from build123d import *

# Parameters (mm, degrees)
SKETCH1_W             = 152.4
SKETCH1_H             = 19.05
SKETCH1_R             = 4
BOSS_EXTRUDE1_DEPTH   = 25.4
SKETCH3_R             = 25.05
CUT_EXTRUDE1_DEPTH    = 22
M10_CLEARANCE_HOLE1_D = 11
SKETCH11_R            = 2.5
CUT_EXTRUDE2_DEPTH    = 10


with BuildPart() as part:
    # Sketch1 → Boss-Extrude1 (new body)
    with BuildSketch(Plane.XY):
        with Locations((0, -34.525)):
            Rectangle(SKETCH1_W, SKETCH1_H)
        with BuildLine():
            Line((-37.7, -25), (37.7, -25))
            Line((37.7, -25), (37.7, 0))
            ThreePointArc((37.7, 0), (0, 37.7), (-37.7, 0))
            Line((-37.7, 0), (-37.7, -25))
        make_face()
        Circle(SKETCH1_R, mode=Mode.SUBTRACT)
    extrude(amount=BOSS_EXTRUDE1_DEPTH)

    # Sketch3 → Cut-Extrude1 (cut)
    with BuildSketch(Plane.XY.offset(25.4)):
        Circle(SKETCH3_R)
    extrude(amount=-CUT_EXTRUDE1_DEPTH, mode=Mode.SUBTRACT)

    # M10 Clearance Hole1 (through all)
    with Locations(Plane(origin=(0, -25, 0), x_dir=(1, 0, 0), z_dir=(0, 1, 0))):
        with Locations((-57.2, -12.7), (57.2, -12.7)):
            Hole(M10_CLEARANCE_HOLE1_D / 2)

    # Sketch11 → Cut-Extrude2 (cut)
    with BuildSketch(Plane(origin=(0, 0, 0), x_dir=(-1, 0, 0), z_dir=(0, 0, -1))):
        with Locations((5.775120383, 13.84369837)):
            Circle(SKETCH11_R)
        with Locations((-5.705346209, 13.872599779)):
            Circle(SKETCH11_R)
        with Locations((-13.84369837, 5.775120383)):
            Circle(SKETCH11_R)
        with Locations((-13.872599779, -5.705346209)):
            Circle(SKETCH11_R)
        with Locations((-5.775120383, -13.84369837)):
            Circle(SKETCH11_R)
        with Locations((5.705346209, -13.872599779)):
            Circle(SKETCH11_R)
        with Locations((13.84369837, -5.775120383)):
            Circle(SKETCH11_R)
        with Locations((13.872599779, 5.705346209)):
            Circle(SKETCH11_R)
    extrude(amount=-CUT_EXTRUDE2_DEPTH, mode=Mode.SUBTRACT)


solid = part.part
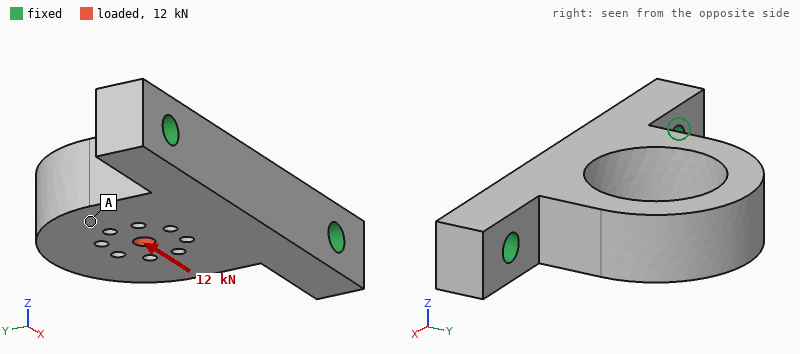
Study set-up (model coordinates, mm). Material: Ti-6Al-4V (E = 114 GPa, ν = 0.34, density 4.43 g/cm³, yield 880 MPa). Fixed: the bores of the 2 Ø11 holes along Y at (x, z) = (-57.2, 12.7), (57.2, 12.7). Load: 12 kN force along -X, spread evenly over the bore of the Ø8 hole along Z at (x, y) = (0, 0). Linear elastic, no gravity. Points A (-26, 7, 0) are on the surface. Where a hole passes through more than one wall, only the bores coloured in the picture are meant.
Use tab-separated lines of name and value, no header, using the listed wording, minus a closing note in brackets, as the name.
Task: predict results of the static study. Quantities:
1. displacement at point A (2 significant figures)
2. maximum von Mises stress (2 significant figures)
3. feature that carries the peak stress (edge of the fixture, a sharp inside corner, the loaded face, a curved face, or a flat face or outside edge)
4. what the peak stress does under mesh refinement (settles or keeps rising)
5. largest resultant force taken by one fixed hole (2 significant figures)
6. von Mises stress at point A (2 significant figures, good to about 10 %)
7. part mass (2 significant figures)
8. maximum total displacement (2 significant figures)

displacement at point A	32 µm
maximum von Mises stress	260 MPa
feature that carries the peak stress	a curved face
what the peak stress does under mesh refinement	settles
largest resultant force taken by one fixed hole	7.6 kN
von Mises stress at point A	20 MPa
part mass	580 g
maximum total displacement	48 µm
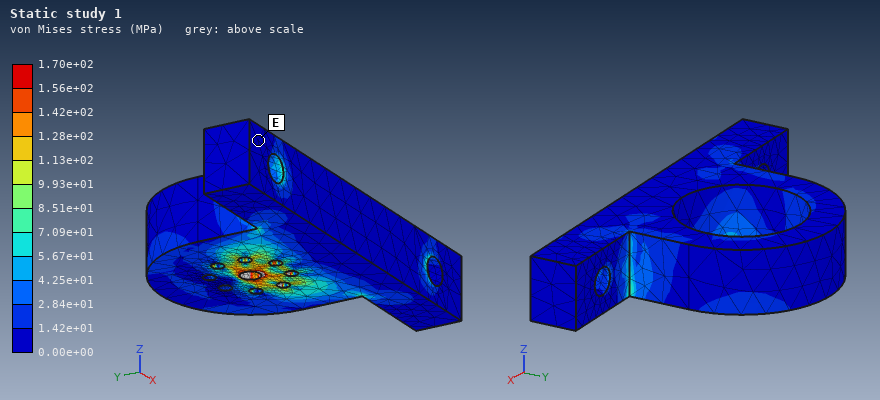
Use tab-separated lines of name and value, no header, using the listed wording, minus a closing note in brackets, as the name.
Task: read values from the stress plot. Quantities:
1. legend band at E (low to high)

legend band at E	0.00e+00 to 1.42e+01 MPa
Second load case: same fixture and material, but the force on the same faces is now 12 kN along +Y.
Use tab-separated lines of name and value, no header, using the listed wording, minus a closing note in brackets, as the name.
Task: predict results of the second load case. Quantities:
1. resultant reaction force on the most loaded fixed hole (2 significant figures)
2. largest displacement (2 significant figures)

resultant reaction force on the most loaded fixed hole	6.4 kN
largest displacement	0.12 mm
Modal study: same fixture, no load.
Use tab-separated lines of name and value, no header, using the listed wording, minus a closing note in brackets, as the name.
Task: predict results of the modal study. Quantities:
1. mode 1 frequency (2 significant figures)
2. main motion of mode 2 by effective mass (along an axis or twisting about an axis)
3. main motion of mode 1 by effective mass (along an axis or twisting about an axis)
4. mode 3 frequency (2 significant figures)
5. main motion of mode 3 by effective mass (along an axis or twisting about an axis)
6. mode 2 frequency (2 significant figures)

mode 1 frequency	2000 Hz
main motion of mode 2 by effective mass	along X
main motion of mode 1 by effective mass	along Z
mode 3 frequency	6300 Hz
main motion of mode 3 by effective mass	along Y
mode 2 frequency	5000 Hz
